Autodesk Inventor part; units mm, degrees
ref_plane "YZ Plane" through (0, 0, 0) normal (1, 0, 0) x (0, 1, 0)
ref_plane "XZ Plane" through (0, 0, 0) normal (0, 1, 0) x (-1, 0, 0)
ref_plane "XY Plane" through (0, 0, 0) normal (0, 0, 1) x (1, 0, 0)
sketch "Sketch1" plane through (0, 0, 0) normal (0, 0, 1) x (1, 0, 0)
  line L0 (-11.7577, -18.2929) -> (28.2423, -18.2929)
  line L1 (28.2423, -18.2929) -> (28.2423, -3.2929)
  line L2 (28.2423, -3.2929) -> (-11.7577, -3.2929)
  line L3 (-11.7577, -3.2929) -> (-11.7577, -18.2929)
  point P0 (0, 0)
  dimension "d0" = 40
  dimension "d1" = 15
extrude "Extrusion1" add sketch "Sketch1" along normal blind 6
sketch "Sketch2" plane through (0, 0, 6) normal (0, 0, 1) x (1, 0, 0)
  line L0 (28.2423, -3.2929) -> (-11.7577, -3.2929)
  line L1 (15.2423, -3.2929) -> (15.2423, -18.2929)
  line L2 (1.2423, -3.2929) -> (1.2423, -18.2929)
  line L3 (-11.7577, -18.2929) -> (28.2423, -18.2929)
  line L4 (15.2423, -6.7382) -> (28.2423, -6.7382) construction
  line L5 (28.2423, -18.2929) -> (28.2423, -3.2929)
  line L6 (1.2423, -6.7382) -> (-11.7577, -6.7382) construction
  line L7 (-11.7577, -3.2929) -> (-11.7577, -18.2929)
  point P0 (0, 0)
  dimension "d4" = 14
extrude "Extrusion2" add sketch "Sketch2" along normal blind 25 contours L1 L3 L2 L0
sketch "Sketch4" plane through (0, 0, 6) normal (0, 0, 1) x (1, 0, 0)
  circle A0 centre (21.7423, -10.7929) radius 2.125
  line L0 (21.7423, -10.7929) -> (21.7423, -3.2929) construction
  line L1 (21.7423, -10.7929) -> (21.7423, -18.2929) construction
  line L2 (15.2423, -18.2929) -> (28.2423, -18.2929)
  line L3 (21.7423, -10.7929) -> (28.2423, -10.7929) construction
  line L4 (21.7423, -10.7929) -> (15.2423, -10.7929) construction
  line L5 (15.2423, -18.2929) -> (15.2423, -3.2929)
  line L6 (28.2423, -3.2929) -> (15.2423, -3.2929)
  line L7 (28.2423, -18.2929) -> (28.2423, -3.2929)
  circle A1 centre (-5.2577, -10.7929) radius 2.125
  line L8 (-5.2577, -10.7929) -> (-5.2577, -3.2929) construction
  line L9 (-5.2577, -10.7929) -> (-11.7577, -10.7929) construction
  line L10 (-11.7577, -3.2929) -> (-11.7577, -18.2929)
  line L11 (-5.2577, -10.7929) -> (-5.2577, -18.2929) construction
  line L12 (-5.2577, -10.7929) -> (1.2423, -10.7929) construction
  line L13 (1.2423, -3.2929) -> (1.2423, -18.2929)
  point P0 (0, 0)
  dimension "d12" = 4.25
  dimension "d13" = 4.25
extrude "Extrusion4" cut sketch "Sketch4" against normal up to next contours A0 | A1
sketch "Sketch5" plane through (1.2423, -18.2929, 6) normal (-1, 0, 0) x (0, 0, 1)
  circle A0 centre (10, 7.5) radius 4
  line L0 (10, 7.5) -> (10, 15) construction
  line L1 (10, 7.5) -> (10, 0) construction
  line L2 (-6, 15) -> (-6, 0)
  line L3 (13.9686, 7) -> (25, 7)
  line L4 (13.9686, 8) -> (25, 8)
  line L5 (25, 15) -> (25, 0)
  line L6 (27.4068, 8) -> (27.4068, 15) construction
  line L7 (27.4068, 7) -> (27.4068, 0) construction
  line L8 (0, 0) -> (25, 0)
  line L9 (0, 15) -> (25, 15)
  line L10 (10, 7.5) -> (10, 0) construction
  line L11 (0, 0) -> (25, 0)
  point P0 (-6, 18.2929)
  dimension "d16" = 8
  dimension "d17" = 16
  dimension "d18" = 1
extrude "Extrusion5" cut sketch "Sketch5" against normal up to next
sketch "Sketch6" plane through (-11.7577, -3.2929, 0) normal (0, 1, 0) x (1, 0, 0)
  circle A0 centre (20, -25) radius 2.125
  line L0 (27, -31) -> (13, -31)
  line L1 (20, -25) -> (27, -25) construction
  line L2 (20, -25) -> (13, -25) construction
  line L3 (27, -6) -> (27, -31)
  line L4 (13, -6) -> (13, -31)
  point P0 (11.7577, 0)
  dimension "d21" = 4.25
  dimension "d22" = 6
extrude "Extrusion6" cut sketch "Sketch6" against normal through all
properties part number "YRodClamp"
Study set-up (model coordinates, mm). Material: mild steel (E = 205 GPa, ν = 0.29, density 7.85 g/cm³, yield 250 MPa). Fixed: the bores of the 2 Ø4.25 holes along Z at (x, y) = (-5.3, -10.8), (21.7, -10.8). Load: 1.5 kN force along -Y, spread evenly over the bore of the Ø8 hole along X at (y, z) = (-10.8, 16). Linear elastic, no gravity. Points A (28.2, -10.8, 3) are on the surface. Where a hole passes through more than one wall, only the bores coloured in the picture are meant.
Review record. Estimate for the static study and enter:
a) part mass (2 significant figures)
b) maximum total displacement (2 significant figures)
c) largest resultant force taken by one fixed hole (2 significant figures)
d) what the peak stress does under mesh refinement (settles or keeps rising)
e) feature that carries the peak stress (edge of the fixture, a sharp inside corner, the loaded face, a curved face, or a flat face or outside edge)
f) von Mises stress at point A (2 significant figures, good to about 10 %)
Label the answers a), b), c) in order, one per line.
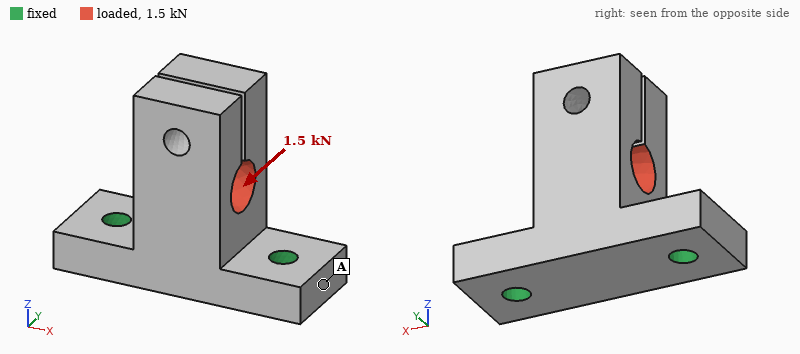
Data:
a) 60 g
b) 46 µm
c) 750 N
d) keeps rising
e) edge of the fixture
f) 21 MPa
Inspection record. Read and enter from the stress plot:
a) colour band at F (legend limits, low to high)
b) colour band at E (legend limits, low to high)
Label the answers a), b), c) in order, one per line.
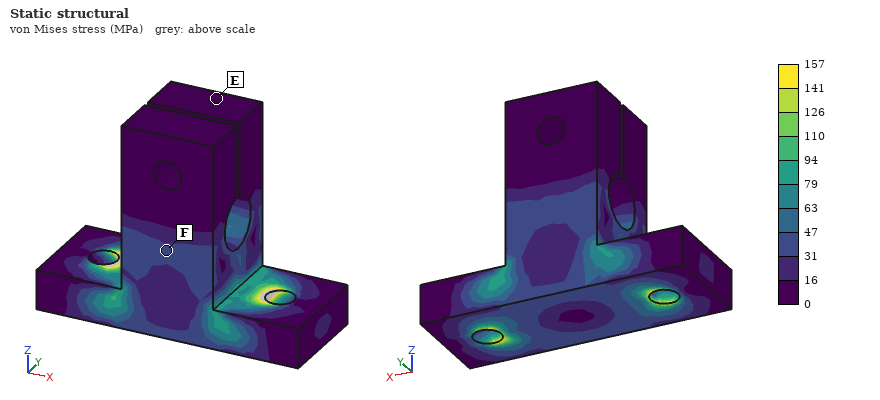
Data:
a) 31 to 47 MPa
b) 0 to 16 MPa
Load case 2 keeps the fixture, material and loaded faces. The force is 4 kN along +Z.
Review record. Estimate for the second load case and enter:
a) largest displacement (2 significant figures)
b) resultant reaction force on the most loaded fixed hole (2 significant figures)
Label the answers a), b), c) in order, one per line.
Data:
a) 31 µm
b) 2.1 kN
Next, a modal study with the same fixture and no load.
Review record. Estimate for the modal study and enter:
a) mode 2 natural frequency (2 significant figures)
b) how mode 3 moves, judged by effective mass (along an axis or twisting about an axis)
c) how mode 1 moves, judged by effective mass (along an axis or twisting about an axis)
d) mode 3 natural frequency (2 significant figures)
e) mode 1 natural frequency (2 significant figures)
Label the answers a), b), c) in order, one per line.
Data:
a) 6200 Hz
b) along X
c) along Y
d) 9900 Hz
e) 4700 Hz
